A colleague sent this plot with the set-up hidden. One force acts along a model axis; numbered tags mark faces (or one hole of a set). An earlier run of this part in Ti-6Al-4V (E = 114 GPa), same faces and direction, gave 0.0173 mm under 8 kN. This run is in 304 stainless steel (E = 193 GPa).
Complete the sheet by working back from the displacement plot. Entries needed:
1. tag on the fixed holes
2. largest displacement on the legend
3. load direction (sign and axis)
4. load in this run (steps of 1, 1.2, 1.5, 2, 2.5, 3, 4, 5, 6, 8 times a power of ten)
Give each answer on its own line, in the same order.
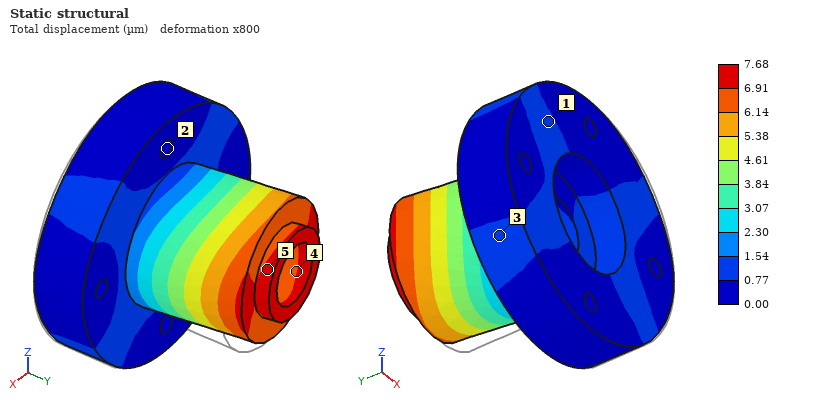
2
7.68 µm
-X
6 kN
